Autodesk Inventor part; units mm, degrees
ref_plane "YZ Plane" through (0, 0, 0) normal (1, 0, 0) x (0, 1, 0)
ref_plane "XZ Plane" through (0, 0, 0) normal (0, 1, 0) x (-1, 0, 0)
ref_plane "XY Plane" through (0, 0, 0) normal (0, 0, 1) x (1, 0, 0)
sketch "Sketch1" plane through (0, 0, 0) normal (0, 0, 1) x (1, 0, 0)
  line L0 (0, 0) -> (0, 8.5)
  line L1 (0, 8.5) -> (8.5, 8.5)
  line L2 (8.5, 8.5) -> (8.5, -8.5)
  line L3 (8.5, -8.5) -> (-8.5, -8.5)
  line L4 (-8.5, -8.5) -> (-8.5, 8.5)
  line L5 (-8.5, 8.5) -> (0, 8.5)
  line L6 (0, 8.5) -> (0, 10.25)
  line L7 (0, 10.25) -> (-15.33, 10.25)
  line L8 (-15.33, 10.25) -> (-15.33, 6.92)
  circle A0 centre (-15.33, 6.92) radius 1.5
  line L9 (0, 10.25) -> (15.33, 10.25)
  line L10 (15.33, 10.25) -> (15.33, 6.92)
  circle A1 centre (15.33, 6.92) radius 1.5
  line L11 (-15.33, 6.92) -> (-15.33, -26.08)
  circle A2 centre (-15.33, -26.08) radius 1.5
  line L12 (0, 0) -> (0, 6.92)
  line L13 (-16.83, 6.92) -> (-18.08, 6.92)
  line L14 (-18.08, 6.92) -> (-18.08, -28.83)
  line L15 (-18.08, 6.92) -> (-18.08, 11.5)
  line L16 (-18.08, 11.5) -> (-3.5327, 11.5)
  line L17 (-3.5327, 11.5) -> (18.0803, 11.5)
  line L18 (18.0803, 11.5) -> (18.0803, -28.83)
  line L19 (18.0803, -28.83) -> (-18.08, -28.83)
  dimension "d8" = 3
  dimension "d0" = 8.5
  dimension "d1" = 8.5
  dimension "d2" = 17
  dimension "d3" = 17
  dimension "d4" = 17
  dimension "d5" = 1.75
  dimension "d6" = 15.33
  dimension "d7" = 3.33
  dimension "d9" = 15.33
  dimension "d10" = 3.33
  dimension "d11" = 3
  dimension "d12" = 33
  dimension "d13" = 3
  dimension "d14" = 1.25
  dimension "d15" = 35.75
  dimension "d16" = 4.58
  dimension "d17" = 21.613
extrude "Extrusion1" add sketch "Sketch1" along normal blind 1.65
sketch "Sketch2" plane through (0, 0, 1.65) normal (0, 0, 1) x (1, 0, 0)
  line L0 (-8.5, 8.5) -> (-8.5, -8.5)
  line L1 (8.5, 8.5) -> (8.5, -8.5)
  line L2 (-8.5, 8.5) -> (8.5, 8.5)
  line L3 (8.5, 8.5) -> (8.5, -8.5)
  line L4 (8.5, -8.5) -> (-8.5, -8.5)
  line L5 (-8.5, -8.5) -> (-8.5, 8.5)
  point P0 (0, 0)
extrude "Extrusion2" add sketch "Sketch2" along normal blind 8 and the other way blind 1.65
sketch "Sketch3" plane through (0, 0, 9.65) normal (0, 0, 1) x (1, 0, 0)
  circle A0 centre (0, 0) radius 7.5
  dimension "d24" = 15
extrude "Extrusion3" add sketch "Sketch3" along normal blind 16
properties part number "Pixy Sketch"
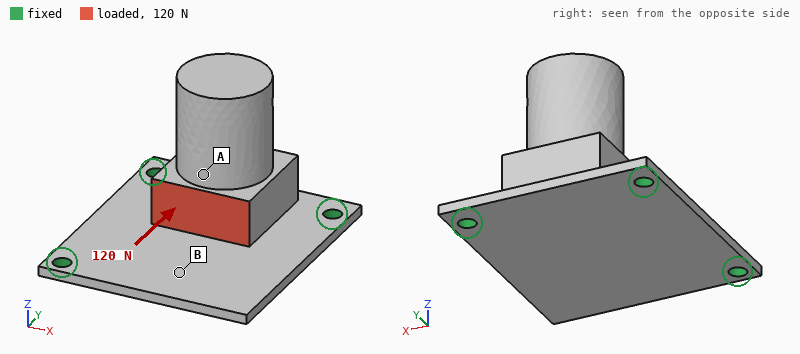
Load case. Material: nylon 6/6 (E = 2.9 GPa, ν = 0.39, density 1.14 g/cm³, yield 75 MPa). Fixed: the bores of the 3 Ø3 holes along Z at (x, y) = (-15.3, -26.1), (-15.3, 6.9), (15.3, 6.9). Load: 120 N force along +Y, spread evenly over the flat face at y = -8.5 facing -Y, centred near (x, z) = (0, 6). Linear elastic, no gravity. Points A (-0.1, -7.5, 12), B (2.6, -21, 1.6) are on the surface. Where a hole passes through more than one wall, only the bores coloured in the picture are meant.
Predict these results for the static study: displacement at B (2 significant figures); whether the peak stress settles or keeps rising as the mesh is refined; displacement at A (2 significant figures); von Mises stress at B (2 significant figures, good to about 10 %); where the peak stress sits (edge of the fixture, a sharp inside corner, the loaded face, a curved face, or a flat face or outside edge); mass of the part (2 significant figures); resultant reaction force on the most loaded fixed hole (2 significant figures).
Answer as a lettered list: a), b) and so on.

a) 0.37 mm
b) keeps rising
c) 0.40 mm
d) 4.5 MPa
e) edge of the fixture
f) 8.6 g
g) 52 N
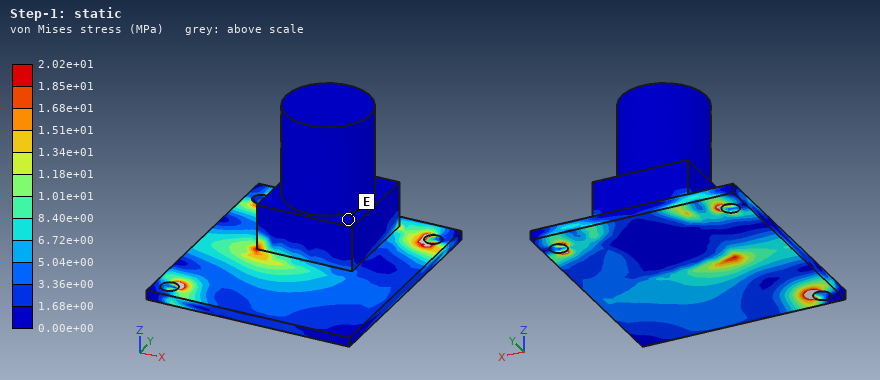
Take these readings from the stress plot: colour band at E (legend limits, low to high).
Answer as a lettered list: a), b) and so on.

a) 0.00e+00 to 1.68e+00 MPa
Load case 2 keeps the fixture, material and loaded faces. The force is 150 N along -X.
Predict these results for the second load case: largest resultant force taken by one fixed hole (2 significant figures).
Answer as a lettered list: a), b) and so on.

a) 77 N
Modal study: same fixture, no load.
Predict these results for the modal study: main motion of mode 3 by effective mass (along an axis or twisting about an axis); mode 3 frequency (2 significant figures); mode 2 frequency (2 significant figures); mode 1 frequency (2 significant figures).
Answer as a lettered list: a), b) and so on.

a) along X
b) 1500 Hz
c) 1200 Hz
d) 590 Hz
